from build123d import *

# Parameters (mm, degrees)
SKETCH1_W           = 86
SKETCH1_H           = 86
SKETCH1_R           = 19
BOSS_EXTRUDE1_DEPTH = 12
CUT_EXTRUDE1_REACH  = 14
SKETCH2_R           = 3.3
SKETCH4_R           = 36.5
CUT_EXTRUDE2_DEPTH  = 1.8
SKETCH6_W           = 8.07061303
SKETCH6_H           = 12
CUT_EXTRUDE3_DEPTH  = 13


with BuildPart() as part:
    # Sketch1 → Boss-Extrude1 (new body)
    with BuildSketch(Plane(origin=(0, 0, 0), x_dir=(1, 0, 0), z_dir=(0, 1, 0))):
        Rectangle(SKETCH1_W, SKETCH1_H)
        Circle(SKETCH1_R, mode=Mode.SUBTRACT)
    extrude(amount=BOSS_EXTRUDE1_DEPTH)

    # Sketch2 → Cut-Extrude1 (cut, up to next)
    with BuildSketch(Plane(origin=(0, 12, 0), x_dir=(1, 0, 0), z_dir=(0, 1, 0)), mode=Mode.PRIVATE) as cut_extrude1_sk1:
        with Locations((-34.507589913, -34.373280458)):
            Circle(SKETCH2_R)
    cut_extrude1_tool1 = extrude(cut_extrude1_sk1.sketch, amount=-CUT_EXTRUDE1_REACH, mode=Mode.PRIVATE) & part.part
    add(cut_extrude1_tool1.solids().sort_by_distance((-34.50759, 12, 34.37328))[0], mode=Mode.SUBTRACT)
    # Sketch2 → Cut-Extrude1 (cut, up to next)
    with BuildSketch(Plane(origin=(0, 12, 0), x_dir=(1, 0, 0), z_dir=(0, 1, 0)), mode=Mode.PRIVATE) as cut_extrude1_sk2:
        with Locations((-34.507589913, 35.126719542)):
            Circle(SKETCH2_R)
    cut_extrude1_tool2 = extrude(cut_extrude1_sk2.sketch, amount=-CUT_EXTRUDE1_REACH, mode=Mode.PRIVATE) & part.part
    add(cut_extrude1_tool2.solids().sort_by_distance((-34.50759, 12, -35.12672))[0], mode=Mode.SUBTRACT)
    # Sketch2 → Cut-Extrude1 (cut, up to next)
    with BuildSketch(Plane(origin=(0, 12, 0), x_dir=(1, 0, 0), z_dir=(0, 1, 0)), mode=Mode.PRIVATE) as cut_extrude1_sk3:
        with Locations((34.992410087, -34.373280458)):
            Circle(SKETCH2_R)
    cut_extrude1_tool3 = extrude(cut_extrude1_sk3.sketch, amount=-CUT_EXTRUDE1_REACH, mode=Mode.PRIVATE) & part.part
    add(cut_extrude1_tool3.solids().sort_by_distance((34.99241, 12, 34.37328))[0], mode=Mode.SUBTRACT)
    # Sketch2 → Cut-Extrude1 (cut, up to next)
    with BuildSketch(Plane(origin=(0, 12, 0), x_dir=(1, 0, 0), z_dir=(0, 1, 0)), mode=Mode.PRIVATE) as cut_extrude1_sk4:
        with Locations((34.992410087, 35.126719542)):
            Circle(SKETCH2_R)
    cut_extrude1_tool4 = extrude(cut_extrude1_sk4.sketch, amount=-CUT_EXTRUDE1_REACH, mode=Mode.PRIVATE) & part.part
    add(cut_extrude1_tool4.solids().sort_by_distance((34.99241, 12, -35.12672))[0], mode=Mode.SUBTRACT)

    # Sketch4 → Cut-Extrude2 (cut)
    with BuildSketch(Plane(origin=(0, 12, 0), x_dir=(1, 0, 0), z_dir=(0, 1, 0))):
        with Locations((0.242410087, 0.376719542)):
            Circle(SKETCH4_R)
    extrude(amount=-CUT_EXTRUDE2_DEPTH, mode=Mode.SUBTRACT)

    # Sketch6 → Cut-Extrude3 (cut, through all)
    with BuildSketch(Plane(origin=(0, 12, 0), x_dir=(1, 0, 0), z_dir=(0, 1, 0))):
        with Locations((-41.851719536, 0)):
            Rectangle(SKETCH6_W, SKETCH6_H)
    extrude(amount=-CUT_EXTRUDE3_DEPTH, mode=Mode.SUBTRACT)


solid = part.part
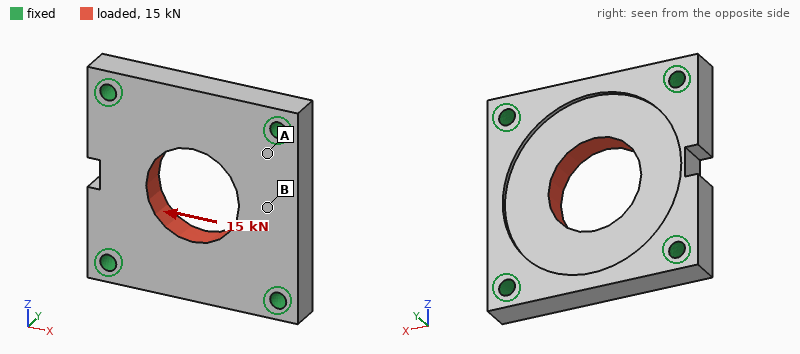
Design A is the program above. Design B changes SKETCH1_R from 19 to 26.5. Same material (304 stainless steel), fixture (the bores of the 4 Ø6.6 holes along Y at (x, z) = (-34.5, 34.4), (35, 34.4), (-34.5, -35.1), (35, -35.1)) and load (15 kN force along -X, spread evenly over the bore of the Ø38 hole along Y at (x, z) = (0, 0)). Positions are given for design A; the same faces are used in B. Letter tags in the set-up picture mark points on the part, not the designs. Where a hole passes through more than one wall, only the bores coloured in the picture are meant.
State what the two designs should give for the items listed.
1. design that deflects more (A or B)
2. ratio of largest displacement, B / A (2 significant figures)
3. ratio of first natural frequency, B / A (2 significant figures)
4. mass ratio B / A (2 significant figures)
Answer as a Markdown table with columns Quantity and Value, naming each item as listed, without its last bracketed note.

| Quantity | Value |
|---|---|
| design that deflects more | B |
| ratio of largest displacement, B / A | 1.5 |
| ratio of first natural frequency, B / A | 1.3 |
| mass ratio B / A | 0.84 |
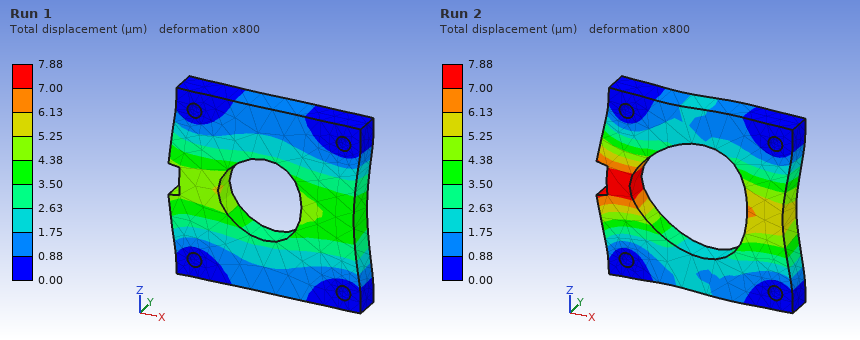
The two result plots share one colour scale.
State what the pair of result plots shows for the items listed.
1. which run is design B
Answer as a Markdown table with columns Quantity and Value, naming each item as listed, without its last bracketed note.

| Quantity | Value |
|---|---|
| which run is design B | Run 2 |
